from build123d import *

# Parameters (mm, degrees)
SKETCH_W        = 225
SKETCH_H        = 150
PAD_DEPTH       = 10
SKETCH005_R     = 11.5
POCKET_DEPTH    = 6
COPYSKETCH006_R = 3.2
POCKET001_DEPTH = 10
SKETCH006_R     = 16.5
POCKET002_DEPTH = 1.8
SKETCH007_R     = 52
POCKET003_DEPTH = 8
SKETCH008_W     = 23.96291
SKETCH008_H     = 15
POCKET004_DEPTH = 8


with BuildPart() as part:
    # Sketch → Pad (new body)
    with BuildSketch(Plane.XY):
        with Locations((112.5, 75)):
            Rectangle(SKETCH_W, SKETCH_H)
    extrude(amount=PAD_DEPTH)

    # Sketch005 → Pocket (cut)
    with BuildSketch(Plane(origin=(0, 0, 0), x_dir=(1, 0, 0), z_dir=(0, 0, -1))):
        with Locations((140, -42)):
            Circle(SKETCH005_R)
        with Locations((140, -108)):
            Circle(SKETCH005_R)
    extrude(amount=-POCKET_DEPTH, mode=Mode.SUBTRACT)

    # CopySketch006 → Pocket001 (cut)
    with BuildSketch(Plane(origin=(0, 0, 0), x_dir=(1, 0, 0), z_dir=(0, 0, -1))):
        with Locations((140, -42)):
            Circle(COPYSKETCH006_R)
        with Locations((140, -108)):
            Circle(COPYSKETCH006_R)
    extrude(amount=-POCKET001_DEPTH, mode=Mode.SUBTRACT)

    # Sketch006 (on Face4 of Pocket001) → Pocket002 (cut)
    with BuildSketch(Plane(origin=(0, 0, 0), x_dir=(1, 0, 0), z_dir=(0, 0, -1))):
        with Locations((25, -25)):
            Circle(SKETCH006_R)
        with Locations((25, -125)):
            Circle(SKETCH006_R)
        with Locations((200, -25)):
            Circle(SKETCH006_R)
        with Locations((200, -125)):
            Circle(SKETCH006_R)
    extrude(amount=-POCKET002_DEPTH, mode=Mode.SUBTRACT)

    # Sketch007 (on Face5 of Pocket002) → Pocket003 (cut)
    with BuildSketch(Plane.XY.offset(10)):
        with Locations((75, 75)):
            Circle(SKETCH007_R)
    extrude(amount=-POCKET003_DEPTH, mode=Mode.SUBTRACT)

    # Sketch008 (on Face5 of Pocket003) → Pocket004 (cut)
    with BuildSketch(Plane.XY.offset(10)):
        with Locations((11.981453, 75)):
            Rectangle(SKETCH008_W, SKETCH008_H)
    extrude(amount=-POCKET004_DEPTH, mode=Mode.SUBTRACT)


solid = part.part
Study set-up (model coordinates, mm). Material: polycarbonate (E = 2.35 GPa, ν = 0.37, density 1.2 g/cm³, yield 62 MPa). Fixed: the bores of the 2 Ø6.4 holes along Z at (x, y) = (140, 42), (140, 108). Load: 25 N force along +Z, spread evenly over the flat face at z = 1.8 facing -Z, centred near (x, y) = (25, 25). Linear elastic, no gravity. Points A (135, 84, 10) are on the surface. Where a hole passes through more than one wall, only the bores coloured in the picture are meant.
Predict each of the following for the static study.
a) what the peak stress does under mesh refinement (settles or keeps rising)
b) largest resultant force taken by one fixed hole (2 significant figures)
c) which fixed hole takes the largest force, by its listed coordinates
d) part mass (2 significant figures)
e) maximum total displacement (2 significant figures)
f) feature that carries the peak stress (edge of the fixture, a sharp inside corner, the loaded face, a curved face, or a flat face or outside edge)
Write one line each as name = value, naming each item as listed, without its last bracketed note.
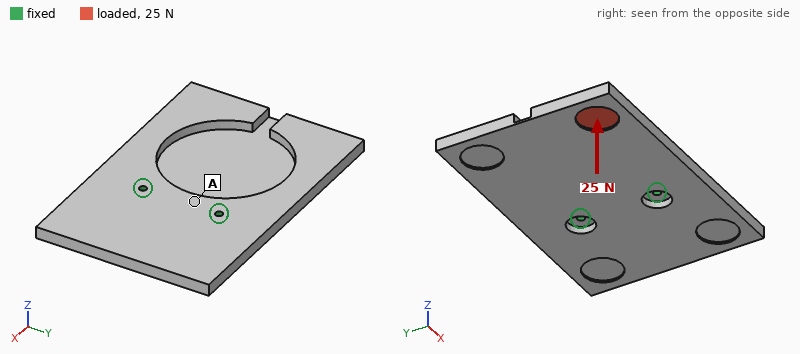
what the peak stress does under mesh refinement = keeps rising
largest resultant force taken by one fixed hole = 35 N
which fixed hole takes the largest force, by its listed coordinates = (140, 42)
part mass = 310 g
maximum total displacement = 2.7 mm
feature that carries the peak stress = edge of the fixture
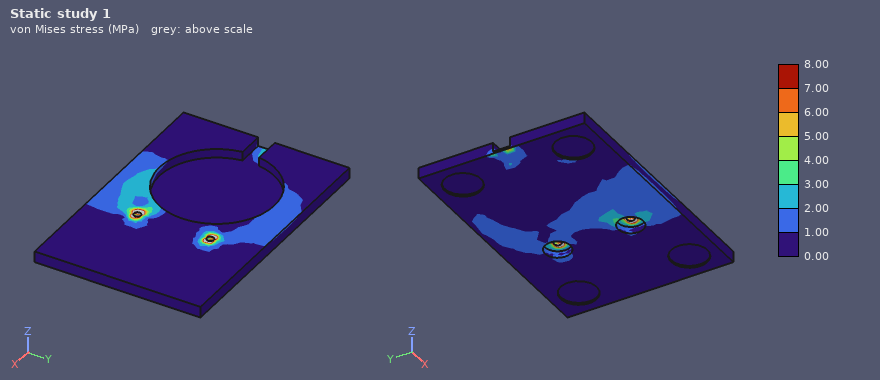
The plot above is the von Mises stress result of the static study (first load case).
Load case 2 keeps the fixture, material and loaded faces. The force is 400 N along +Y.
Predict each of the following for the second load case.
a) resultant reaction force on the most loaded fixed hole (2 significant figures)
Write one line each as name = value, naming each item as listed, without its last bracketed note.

resultant reaction force on the most loaded fixed hole = 700 N
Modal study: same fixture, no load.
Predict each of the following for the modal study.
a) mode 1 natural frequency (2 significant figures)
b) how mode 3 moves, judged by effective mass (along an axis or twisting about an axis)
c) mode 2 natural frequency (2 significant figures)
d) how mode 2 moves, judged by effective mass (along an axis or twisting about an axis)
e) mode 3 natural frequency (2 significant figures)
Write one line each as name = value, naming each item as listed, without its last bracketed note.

mode 1 natural frequency = 62 Hz
how mode 3 moves, judged by effective mass = along Z
mode 2 natural frequency = 160 Hz
how mode 2 moves, judged by effective mass = twisting about X
mode 3 natural frequency = 190 Hz
